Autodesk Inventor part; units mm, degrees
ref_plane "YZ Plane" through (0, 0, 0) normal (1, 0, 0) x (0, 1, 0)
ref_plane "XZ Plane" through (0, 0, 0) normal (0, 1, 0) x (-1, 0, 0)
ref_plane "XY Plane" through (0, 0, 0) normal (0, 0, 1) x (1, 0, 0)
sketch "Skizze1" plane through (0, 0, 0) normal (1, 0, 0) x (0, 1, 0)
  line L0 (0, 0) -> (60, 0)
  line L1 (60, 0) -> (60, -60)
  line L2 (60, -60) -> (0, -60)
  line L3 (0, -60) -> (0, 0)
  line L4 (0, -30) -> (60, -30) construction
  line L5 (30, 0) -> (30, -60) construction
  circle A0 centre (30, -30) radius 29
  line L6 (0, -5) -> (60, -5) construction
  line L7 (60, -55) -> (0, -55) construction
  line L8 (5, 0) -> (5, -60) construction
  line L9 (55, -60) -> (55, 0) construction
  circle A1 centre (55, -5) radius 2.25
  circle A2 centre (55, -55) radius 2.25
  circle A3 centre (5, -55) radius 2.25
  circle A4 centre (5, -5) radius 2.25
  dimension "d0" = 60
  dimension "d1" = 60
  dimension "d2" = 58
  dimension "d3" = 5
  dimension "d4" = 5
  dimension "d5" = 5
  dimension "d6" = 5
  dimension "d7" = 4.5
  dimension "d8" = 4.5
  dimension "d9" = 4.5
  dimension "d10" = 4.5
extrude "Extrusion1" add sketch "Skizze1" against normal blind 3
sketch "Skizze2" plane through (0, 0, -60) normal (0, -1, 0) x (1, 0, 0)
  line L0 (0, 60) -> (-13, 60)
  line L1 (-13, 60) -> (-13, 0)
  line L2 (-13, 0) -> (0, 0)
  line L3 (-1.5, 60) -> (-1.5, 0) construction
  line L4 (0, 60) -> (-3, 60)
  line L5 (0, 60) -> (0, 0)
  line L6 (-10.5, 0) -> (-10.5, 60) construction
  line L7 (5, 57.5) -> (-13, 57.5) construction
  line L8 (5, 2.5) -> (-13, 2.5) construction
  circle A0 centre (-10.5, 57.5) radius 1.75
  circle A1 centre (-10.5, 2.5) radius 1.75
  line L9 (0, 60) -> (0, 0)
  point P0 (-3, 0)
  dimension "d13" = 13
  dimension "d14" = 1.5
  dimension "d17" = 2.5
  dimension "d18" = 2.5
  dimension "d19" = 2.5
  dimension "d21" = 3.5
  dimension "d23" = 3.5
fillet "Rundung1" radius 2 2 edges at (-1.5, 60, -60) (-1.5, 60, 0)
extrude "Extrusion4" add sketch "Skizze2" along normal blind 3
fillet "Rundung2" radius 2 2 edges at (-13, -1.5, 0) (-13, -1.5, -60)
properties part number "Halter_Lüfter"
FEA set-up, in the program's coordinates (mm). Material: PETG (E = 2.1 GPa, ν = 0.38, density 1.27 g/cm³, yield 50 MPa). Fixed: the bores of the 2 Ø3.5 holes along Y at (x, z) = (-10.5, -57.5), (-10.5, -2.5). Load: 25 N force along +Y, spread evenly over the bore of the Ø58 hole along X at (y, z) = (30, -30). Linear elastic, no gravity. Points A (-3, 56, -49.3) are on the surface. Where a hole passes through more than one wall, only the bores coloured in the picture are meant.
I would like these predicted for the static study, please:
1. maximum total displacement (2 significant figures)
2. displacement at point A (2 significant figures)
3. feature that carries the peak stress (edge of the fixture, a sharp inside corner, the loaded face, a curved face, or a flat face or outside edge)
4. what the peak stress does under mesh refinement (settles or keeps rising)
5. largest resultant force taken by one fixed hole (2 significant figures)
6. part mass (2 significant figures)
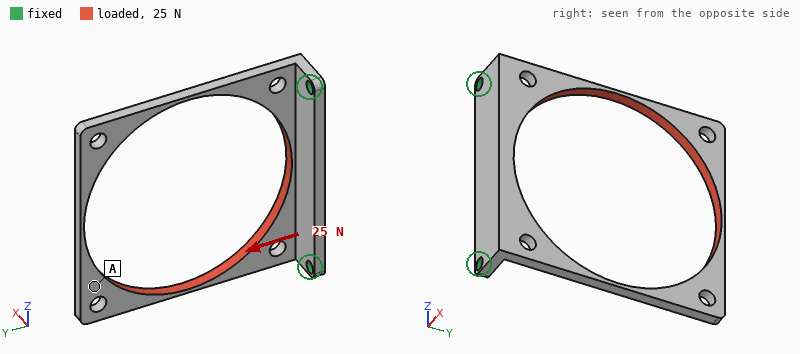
0.89 mm
0.54 mm
a sharp inside corner
keeps rising
13 N
6.3 g
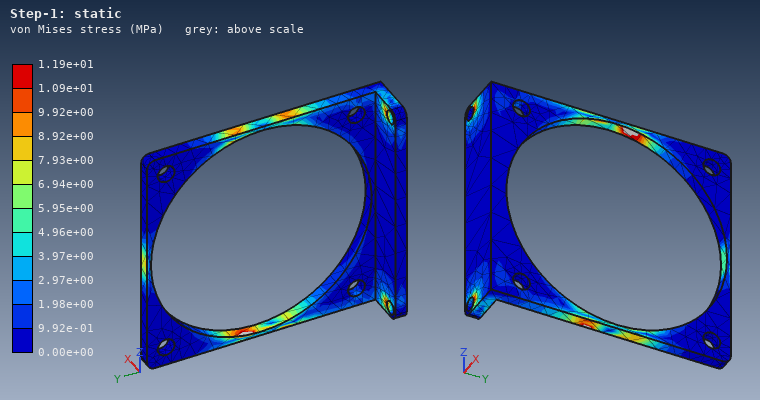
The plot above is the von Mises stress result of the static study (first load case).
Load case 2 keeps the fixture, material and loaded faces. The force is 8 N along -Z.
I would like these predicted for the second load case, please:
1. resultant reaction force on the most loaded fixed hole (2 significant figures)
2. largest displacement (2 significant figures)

6.0 N
0.92 mm
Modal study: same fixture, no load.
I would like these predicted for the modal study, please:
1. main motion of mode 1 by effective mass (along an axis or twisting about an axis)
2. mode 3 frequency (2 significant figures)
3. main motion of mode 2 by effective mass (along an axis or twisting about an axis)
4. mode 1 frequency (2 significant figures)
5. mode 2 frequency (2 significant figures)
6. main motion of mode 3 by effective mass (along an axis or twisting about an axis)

along X
260 Hz
twisting about Y
92 Hz
170 Hz
along Z
